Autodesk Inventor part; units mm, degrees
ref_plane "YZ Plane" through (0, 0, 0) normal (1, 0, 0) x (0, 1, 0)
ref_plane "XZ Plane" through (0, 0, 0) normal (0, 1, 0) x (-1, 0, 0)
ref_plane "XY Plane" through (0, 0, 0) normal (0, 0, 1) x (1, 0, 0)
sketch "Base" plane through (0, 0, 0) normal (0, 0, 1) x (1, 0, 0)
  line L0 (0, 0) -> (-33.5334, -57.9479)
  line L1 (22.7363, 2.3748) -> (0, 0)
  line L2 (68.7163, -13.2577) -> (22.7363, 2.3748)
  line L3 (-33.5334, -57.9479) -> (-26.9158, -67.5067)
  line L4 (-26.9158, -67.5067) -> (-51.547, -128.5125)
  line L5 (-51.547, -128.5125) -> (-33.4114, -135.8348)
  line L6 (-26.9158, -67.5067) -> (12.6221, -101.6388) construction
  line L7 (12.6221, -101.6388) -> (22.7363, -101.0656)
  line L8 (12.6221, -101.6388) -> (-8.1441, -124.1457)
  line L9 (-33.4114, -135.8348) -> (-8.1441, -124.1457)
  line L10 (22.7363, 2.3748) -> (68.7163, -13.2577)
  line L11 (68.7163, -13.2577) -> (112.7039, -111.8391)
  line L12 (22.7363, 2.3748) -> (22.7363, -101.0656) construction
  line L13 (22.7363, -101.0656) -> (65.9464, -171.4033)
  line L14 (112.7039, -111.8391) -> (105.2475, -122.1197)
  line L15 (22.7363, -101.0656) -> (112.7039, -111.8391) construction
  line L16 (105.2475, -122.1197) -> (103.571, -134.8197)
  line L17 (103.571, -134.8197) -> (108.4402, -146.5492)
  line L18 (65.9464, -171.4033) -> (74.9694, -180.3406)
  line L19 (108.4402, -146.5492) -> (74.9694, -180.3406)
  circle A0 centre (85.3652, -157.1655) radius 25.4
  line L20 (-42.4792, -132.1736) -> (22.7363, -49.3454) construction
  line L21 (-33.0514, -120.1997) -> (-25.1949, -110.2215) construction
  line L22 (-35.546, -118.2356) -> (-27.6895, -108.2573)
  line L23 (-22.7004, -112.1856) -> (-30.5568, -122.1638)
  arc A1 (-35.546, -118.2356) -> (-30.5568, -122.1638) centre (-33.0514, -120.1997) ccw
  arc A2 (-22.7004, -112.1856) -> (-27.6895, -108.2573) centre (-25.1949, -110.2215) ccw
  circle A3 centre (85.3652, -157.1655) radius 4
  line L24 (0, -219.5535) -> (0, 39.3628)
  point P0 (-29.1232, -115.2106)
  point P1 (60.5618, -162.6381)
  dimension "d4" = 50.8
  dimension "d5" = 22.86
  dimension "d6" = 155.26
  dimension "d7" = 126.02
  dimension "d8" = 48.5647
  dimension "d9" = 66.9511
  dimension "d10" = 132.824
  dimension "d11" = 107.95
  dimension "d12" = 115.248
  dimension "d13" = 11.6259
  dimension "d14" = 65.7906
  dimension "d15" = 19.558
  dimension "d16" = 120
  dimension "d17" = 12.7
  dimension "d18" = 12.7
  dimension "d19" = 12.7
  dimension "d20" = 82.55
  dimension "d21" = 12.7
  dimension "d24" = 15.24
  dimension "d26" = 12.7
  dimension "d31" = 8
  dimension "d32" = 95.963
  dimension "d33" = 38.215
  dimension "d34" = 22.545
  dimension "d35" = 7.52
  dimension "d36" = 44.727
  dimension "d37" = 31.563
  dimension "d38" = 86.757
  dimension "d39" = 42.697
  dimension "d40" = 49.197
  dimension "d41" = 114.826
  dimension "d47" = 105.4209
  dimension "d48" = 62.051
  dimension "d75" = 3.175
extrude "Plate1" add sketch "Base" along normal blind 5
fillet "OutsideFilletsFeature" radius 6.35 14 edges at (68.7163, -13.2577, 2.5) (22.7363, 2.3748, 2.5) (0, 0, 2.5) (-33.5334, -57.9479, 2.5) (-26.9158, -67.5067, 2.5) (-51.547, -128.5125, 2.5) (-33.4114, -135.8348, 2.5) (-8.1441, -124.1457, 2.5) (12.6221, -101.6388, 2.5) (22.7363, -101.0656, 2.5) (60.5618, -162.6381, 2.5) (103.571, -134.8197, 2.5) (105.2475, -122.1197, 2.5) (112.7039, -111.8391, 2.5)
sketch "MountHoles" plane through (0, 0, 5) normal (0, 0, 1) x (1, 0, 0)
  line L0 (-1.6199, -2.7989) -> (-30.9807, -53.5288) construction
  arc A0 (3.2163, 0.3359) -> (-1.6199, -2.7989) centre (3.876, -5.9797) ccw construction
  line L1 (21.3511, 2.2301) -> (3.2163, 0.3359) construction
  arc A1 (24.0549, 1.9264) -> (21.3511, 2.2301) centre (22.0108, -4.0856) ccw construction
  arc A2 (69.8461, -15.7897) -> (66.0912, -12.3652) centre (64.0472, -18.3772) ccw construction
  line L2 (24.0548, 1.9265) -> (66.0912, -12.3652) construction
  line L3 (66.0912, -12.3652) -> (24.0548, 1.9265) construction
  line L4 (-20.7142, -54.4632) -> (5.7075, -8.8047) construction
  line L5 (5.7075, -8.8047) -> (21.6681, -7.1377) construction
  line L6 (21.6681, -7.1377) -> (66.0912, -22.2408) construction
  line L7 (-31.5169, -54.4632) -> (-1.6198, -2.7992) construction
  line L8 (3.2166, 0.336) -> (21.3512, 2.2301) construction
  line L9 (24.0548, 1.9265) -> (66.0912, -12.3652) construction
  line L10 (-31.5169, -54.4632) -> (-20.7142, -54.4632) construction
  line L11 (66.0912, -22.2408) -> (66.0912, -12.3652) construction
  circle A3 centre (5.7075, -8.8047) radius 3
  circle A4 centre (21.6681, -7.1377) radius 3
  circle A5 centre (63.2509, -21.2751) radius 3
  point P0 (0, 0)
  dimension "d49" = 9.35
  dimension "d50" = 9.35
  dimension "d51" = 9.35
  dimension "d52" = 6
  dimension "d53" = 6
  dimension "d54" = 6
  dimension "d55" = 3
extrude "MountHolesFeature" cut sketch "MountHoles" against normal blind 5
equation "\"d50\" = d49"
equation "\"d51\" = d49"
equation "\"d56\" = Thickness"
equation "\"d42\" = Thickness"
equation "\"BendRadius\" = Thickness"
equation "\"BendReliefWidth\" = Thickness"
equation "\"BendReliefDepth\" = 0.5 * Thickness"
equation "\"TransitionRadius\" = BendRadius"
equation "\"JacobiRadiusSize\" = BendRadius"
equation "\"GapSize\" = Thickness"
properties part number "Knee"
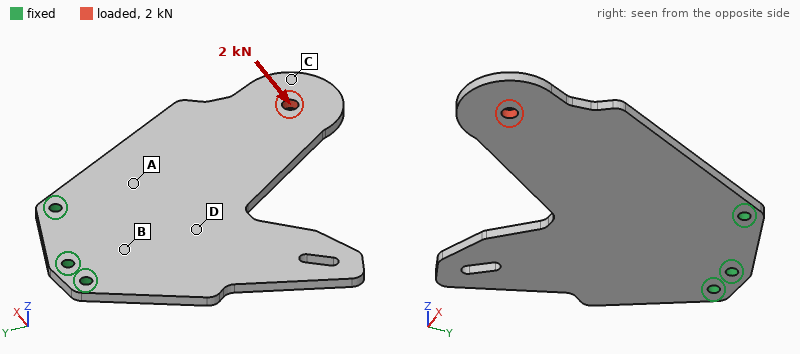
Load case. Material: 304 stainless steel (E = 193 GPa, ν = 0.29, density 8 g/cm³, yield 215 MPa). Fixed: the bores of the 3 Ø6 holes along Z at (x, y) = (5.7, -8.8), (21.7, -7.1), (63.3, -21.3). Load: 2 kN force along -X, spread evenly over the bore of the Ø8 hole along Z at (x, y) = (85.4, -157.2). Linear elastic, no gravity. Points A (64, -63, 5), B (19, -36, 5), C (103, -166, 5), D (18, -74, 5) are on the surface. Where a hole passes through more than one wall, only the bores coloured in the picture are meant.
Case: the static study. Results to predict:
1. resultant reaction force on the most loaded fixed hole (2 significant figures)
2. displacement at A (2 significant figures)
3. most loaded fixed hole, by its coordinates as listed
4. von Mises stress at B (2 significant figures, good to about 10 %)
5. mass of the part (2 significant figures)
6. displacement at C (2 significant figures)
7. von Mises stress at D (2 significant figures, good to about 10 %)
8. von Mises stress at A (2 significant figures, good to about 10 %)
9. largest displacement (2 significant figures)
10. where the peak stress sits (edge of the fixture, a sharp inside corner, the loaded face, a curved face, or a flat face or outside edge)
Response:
5.0 kN
14 µm
(63.3, -21.3)
24 MPa
670 g
71 µm
21 MPa
12 MPa
76 µm
edge of the fixture
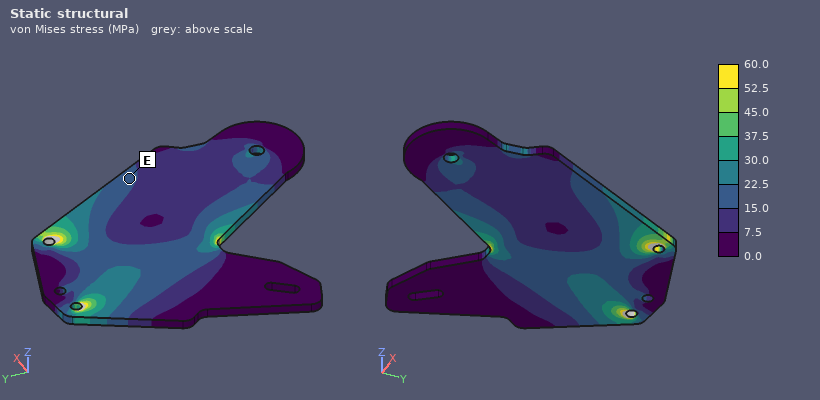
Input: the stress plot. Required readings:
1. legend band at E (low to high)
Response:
15.0 to 22.5 MPa
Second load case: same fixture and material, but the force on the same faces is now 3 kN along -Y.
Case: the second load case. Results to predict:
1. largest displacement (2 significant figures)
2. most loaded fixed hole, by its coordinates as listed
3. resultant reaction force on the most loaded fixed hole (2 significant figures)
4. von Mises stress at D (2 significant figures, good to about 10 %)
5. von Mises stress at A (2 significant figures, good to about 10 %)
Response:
41 µm
(63.3, -21.3)
3.9 kN
6.4 MPa
15 MPa
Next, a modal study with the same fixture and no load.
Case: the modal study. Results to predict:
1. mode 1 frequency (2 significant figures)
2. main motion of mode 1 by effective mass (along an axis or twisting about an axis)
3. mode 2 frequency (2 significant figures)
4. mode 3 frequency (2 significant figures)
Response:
170 Hz
along Z
380 Hz
980 Hz
